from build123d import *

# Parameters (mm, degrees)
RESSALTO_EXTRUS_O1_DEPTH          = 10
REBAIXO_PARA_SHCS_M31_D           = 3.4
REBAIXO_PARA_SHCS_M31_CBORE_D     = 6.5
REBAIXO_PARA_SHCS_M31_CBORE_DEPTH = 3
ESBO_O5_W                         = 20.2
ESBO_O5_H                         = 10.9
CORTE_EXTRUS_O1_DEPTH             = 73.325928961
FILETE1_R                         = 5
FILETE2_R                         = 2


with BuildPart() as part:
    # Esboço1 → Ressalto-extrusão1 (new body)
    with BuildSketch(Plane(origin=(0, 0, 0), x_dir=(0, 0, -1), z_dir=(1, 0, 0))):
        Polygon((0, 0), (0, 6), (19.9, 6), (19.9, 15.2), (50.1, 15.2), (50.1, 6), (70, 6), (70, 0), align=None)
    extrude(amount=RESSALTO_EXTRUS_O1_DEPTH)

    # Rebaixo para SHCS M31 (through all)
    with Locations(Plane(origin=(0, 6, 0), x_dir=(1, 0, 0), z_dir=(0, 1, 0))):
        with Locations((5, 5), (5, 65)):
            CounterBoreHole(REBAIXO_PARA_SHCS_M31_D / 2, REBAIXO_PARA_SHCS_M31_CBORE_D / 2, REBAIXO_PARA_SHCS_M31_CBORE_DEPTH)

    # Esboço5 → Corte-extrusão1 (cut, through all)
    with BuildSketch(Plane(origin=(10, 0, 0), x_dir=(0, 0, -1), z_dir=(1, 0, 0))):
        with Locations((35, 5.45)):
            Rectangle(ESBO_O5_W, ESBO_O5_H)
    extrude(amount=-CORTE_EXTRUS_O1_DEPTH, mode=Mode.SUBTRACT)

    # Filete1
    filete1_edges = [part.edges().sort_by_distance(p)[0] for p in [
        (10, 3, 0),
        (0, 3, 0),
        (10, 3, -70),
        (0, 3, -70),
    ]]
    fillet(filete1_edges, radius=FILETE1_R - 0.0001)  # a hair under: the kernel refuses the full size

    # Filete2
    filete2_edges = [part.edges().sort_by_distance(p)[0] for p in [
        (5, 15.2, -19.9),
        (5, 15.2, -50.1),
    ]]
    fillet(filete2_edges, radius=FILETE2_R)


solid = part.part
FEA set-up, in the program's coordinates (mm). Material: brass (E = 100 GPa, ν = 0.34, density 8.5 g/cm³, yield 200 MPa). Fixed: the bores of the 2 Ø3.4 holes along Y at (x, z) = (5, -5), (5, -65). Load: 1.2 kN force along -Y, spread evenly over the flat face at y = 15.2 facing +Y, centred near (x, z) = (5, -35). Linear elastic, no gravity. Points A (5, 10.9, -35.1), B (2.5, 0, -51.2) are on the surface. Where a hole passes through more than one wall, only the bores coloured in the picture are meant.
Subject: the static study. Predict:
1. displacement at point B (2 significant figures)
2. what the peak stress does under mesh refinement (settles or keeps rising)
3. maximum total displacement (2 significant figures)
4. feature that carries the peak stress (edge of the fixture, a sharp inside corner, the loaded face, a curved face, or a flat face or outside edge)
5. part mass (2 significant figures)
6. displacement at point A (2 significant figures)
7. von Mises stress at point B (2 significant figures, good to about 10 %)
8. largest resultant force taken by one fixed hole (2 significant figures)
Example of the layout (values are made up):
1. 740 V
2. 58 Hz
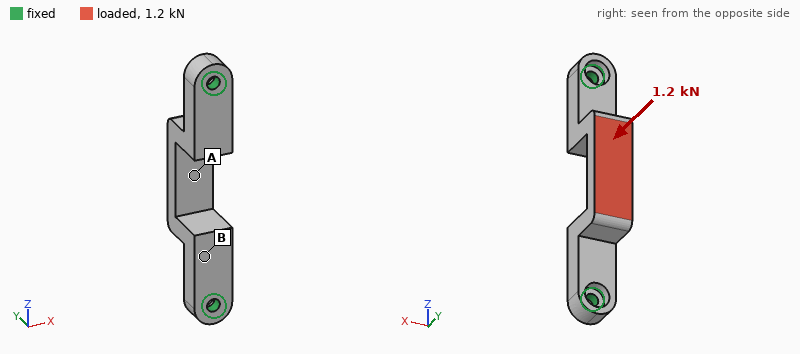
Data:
1. 29 µm
2. keeps rising
3. 41 µm
4. edge of the fixture
5. 37 g
6. 40 µm
7. 33 MPa
8. 1.0 kN
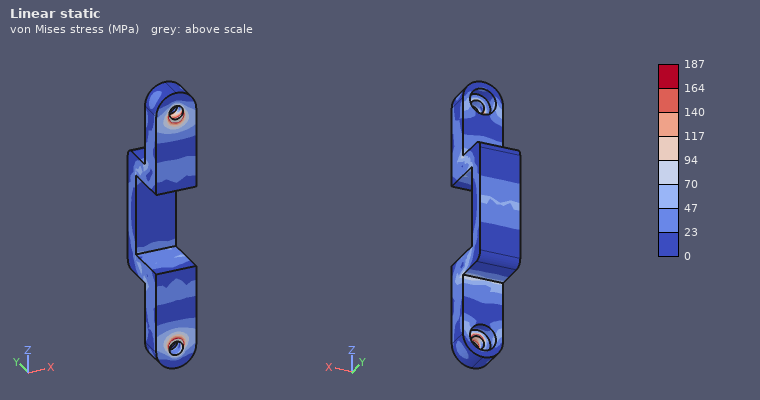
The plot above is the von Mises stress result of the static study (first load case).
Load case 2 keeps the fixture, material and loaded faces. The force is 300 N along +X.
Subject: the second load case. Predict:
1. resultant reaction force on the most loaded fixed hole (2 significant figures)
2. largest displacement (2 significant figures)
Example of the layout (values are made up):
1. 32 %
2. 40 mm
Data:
1. 150 N
2. 51 µm
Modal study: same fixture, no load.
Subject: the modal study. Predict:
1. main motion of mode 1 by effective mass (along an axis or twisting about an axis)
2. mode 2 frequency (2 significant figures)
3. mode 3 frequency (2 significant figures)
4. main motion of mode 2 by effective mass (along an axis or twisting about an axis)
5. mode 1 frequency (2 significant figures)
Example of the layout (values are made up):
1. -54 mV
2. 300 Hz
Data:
1. along X
2. 5900 Hz
3. 6900 Hz
4. along Y
5. 3700 Hz
